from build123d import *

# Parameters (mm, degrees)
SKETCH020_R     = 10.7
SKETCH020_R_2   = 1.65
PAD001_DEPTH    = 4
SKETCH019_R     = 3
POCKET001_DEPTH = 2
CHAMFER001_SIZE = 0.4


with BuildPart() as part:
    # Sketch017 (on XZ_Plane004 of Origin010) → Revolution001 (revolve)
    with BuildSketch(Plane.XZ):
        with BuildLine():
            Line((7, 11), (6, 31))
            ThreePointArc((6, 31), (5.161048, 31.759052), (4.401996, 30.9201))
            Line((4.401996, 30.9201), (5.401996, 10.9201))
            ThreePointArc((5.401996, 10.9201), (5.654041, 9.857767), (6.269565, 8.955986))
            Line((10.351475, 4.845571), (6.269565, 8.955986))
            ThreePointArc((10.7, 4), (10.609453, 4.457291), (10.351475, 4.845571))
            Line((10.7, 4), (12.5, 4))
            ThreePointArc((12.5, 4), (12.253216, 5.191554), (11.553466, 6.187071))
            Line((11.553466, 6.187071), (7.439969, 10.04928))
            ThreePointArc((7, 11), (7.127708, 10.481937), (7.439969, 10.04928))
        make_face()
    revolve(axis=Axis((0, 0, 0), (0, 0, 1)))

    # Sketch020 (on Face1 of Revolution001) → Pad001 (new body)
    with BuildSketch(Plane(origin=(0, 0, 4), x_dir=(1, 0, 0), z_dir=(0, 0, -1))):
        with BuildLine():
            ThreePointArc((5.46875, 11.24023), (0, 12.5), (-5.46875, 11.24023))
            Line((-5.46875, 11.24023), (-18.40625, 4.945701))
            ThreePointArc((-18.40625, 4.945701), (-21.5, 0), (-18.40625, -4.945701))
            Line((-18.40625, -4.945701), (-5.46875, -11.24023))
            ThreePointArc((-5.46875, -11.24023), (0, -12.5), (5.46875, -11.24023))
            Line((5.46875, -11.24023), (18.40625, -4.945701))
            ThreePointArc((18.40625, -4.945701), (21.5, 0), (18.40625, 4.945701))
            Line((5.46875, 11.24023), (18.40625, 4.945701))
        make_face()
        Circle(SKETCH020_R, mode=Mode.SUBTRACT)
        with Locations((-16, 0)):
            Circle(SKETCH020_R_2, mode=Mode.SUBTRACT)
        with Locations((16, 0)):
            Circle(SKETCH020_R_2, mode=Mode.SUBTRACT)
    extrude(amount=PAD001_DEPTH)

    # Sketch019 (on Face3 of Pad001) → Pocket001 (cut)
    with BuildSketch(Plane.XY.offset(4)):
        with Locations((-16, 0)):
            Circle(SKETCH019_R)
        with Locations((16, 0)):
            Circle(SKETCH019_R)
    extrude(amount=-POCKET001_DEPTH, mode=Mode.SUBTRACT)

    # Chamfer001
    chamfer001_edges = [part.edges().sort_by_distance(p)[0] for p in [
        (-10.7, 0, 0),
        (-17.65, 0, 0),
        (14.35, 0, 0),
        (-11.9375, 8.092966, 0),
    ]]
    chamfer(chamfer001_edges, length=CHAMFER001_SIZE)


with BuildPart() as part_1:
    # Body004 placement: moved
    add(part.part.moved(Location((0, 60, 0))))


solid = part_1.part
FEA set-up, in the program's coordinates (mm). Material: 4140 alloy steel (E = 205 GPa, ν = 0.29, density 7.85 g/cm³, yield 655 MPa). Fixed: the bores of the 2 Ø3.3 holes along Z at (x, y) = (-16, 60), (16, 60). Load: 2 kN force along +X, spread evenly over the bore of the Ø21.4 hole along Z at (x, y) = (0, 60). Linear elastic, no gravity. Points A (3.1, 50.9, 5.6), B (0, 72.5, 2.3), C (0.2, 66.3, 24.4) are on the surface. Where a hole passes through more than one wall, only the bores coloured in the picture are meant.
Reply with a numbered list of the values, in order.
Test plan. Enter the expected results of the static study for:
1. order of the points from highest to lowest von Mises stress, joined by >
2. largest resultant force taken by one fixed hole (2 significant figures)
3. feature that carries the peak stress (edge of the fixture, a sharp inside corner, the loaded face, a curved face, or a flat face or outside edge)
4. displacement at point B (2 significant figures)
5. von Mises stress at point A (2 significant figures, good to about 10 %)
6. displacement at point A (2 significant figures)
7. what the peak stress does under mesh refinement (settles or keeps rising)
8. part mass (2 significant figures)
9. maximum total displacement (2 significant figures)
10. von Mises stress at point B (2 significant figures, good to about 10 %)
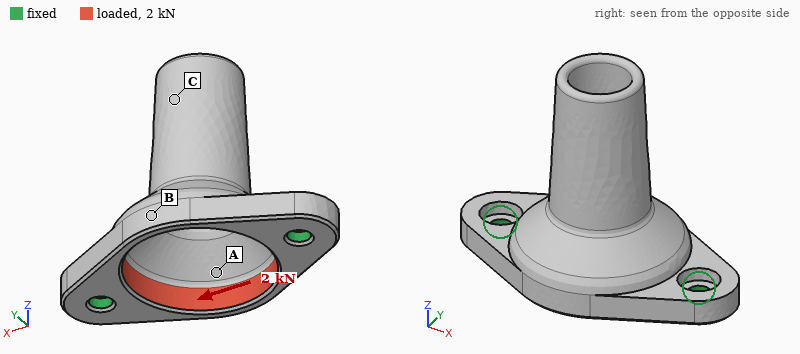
1. B > A > C
2. 1.0 kN
3. edge of the fixture
4. 4.0 µm
5. 24 MPa
6. 3.8 µm
7. keeps rising
8. 26 g
9. 7.7 µm
10. 44 MPa
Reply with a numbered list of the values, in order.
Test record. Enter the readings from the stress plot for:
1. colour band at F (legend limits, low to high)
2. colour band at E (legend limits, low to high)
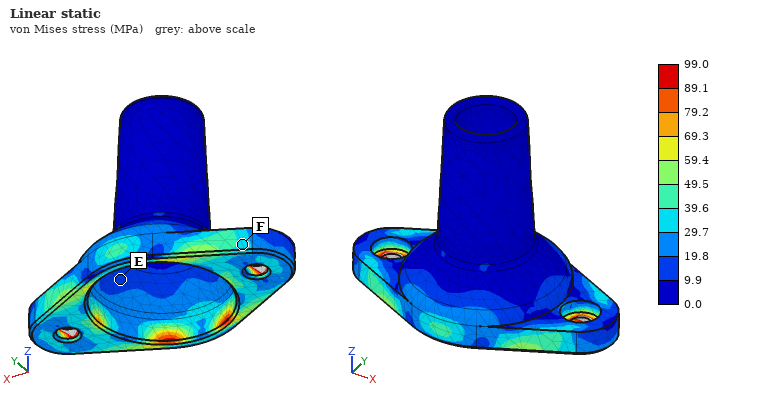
1. 29.7 to 39.6 MPa
2. 9.9 to 19.8 MPa
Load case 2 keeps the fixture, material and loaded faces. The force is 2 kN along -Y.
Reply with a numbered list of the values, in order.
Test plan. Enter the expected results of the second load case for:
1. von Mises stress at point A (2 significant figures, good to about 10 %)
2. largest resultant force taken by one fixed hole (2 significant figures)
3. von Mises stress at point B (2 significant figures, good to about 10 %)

1. 19 MPa
2. 1.0 kN
3. 35 MPa
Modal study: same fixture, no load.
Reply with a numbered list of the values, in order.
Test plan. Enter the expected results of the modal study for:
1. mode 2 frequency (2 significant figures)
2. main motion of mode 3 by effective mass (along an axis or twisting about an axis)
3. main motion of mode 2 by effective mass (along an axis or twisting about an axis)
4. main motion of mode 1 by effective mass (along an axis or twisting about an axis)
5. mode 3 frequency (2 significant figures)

1. 12 kHz
2. along Z
3. along X
4. along Y
5. 15 kHz
